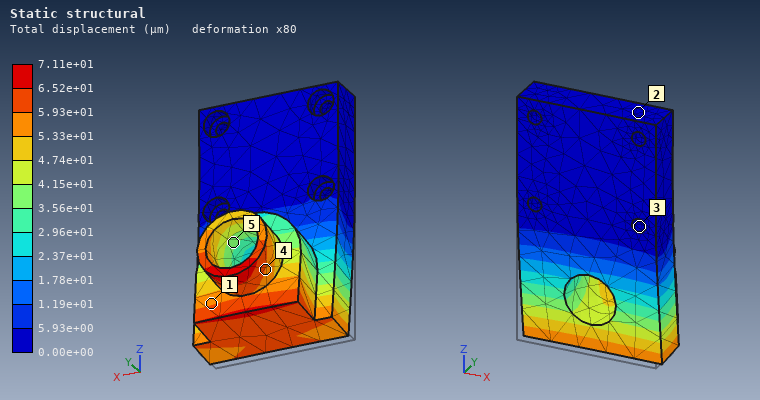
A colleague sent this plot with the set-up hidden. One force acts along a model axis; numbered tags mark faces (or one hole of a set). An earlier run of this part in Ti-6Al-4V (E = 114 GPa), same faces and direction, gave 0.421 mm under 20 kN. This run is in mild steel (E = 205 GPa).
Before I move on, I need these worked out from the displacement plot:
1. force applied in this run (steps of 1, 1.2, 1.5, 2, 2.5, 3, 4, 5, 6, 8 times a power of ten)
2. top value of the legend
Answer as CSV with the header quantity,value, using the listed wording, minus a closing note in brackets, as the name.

quantity,value
force applied in this run,6 kN
top value of the legend,7.11e+01 µm
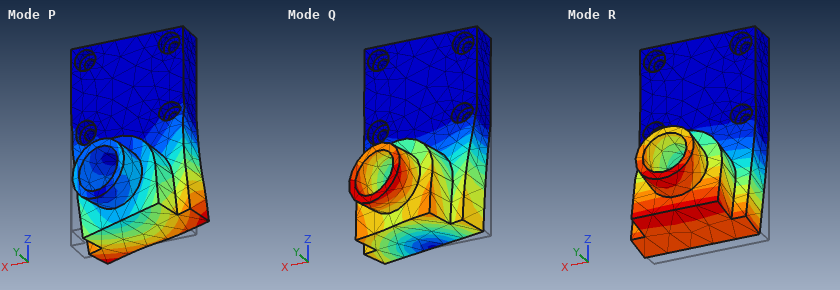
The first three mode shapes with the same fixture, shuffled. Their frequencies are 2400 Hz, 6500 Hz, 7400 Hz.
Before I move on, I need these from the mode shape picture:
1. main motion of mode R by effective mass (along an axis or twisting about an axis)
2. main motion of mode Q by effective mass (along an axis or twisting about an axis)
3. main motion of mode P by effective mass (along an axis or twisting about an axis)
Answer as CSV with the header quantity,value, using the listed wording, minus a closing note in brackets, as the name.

quantity,value
main motion of mode R by effective mass,along Y
main motion of mode Q by effective mass,along X
main motion of mode P by effective mass,along X
